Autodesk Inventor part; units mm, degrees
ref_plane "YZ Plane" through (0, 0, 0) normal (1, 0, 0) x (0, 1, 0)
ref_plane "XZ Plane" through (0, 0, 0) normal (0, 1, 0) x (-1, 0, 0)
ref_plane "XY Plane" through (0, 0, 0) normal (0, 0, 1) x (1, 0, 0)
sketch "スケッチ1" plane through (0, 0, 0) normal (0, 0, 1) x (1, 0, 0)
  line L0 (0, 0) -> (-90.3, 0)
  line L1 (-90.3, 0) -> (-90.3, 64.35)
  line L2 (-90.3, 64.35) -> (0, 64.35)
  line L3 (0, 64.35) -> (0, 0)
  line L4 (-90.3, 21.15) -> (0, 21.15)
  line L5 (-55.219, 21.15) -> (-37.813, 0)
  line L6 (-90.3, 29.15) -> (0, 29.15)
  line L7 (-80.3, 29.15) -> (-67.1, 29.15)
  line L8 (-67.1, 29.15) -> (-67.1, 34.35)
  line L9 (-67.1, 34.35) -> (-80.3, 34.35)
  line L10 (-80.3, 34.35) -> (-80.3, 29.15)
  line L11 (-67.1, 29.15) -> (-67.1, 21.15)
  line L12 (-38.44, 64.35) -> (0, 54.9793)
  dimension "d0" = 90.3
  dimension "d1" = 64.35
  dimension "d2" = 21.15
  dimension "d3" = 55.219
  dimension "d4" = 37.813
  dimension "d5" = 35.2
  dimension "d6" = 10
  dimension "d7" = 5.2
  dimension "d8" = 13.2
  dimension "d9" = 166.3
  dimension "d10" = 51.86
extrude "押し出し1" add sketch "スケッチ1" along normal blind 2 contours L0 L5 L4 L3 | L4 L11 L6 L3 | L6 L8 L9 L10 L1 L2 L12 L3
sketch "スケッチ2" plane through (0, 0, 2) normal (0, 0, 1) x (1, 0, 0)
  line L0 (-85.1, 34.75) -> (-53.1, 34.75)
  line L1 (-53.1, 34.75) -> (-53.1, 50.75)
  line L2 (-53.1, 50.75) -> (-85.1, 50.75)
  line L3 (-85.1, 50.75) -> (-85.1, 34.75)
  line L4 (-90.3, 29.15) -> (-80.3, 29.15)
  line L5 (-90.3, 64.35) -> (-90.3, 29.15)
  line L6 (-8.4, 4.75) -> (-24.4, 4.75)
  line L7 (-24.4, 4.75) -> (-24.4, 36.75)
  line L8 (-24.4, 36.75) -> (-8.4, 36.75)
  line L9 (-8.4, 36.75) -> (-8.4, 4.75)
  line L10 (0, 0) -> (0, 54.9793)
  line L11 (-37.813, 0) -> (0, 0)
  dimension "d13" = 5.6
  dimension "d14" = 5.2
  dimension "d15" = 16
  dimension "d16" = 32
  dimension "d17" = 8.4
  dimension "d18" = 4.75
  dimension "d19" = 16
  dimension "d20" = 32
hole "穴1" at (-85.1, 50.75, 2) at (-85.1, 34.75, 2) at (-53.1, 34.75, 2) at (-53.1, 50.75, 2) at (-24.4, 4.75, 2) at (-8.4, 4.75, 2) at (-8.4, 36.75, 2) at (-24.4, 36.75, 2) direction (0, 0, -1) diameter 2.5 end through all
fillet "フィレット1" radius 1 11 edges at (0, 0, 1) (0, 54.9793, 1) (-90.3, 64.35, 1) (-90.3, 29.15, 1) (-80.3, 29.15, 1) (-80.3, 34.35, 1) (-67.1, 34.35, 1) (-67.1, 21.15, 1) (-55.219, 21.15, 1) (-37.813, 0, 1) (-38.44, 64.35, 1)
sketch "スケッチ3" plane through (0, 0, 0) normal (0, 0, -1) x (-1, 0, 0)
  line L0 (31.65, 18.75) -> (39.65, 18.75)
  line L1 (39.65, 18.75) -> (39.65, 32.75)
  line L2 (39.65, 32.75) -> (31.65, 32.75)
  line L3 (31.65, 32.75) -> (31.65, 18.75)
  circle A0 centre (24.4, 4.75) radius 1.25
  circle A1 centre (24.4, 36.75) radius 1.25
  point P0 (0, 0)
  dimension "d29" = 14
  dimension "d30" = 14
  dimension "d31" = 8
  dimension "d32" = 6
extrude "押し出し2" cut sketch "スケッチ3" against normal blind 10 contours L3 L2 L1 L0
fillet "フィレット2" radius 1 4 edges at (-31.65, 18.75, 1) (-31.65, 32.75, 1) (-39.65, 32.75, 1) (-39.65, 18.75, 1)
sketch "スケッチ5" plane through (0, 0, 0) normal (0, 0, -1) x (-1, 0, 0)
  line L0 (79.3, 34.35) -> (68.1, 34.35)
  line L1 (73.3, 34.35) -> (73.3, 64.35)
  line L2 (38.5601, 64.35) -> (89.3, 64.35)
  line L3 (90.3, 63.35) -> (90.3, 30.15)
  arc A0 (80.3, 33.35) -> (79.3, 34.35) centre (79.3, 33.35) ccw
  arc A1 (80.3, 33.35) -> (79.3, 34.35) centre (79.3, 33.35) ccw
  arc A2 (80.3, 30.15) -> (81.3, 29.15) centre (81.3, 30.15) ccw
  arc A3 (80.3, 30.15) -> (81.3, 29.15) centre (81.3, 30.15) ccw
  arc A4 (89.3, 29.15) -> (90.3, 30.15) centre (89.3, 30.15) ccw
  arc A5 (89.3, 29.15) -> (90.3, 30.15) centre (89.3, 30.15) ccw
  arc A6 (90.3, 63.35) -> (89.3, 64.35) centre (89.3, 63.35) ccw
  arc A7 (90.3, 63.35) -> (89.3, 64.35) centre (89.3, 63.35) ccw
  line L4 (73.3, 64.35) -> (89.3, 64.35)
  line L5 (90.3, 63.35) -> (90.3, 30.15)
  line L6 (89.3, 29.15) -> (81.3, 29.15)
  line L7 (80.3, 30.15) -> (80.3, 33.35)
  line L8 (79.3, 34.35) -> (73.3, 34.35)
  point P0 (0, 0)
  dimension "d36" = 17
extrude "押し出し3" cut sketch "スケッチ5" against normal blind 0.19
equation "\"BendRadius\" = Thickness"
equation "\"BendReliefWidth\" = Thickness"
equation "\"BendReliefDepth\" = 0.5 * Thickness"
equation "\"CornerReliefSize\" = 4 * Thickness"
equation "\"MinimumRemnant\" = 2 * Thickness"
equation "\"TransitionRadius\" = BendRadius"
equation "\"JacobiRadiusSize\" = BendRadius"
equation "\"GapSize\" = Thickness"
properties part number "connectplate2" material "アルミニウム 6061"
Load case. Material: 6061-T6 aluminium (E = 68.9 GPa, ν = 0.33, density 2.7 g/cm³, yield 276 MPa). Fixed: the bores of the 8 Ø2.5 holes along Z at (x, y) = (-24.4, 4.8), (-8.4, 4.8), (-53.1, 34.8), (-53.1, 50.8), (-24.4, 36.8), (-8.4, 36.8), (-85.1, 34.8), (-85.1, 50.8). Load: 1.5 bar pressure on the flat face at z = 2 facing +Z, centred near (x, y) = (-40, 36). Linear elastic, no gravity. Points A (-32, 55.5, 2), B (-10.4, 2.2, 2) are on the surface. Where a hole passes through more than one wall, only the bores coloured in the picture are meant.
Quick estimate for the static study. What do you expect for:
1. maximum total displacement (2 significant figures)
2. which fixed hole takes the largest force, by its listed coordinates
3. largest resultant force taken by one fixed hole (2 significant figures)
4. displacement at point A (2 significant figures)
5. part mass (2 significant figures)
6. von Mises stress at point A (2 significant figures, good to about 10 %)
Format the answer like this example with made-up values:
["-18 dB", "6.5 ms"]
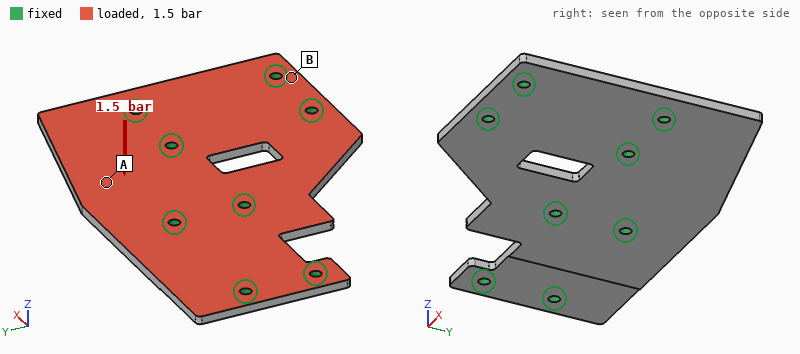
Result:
["81 µm", "(-53.1, 50.8)", "130 N", "49 µm", "23 g", "12 MPa"]
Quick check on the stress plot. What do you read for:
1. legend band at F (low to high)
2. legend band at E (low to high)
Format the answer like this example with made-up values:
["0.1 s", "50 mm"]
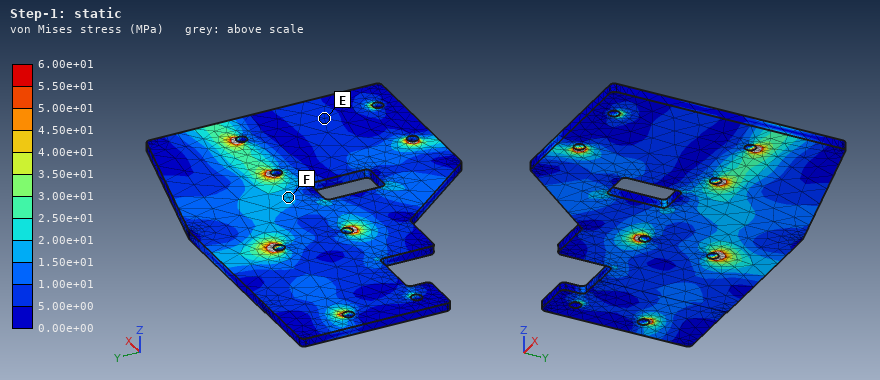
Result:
["1.50e+01 to 2.00e+01 MPa", "5.00e+00 to 1.00e+01 MPa"]
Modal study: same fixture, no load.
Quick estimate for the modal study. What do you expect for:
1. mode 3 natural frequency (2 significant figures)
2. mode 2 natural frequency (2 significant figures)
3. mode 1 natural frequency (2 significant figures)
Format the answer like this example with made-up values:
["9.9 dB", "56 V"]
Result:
["6300 Hz", "5400 Hz", "3800 Hz"]
